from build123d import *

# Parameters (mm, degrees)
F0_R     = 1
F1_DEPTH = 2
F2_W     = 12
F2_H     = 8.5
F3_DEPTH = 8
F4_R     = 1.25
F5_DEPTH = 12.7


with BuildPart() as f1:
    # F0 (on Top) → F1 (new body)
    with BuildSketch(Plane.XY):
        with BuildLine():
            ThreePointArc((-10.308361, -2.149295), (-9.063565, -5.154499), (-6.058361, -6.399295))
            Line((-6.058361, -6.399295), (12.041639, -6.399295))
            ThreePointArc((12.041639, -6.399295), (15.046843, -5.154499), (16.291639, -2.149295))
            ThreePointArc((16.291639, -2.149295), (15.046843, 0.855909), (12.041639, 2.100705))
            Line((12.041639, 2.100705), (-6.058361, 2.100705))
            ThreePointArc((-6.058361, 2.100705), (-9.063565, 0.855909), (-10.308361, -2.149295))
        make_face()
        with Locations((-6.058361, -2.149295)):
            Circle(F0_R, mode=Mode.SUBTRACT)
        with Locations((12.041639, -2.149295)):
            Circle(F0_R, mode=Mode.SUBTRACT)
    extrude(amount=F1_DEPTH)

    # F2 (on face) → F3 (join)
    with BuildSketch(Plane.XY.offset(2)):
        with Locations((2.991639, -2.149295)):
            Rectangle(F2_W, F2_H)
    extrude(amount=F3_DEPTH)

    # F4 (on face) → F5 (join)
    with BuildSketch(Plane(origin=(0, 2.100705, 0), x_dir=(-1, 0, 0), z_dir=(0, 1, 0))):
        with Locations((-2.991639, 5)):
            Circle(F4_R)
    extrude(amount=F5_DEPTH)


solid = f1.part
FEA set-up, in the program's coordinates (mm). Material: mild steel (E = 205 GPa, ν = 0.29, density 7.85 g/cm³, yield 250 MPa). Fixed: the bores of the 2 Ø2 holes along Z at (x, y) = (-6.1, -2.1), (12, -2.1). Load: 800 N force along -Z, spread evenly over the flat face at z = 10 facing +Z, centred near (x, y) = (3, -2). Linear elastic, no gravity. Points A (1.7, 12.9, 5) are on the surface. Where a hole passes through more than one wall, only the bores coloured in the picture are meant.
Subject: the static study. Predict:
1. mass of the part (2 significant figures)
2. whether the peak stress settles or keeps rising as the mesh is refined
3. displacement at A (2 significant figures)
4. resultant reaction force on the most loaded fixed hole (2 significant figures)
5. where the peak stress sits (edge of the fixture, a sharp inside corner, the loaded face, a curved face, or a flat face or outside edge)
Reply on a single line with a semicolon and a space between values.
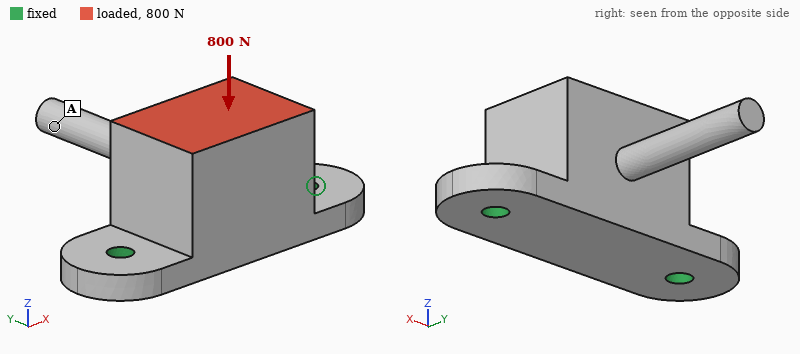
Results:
10 g; keeps rising; 3.9 µm; 440 N; edge of the fixture
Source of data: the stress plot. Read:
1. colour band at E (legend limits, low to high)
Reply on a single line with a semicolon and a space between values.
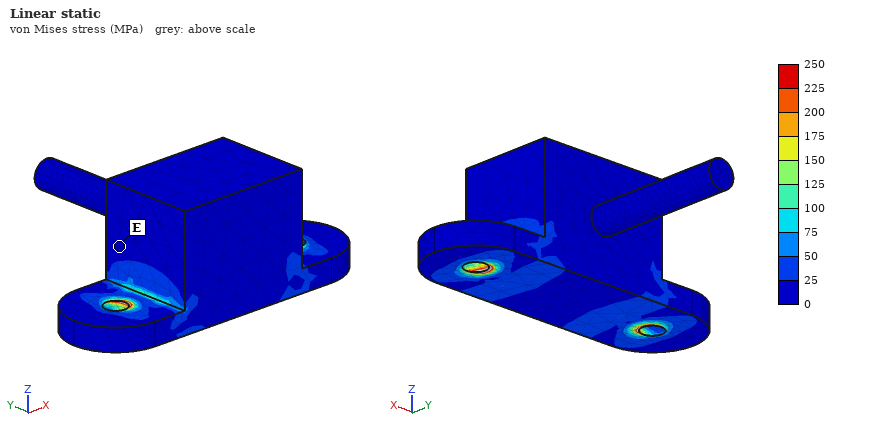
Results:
0 to 25 MPa
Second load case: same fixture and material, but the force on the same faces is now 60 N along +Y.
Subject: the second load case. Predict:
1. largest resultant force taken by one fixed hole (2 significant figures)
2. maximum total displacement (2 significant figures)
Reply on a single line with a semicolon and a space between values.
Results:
30 N; 8.5 µm
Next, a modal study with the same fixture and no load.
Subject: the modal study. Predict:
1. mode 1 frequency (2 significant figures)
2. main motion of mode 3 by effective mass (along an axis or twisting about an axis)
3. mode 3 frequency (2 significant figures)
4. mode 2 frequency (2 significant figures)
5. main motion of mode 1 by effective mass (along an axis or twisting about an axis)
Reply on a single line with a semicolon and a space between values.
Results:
8100 Hz; along Y; 12 kHz; 9900 Hz; along Y
